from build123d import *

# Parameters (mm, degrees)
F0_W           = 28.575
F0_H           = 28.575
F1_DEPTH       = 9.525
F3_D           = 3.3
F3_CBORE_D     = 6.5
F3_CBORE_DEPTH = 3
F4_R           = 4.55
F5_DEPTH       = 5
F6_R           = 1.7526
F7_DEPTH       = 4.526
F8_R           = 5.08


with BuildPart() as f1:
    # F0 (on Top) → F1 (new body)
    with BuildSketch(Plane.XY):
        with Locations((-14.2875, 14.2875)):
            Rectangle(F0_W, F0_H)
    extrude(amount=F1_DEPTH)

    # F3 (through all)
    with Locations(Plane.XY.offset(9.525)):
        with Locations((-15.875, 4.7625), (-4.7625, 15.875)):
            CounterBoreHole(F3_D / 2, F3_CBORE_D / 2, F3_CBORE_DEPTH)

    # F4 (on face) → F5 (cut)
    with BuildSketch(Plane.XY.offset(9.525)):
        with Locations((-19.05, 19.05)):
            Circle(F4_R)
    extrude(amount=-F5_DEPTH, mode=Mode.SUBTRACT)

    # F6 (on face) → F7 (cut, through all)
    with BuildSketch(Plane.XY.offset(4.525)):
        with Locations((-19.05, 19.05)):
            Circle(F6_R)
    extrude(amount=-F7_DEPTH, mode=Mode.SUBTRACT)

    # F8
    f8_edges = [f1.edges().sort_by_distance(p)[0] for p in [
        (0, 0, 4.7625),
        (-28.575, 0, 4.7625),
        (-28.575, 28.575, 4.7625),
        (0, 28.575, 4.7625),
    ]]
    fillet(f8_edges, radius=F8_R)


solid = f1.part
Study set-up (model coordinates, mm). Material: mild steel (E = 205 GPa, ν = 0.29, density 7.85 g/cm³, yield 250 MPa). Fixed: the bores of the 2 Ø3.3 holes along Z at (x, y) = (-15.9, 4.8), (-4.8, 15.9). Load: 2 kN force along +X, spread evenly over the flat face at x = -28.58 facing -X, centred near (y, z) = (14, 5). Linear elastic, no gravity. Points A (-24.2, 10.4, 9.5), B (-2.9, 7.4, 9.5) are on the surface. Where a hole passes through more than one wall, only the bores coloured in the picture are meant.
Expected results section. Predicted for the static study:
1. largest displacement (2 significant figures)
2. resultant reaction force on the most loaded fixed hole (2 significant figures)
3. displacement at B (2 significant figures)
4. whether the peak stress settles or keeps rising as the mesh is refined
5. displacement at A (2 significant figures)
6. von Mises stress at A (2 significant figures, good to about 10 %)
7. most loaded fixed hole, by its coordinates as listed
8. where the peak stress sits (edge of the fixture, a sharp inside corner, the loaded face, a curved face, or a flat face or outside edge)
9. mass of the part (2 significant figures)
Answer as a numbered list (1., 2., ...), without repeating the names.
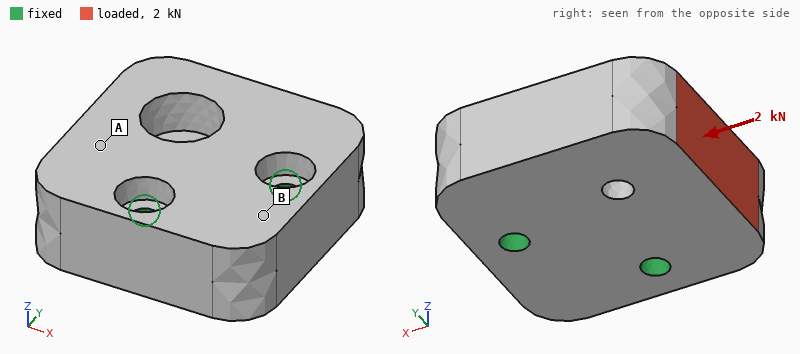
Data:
1. 3.3 µm
2. 1.3 kN
3. 0.51 µm
4. keeps rising
5. 1.7 µm
6. 14 MPa
7. (-4.8, 15.9)
8. edge of the fixture
9. 54 g
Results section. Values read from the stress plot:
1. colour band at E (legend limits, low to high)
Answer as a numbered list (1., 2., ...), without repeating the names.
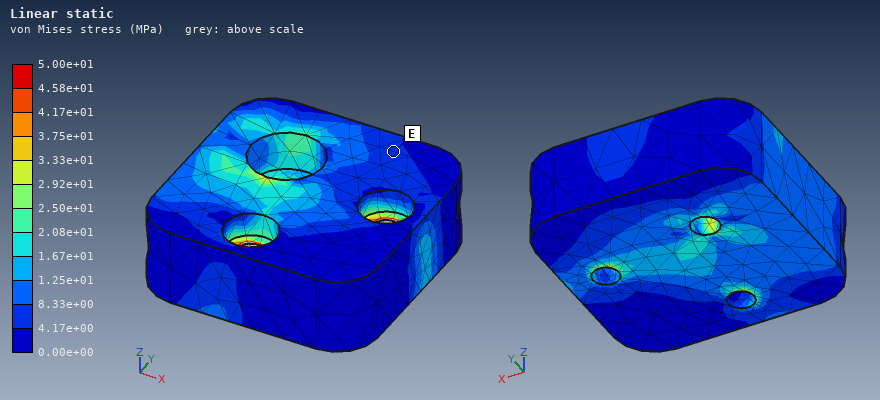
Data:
1. 4.17e+00 to 8.33e+00 MPa
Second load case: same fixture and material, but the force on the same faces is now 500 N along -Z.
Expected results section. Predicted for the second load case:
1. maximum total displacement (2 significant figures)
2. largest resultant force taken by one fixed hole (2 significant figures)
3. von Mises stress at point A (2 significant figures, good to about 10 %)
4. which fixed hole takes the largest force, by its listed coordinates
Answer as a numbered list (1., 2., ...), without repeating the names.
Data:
1. 7.0 µm
2. 490 N
3. 8.5 MPa
4. (-15.9, 4.8)
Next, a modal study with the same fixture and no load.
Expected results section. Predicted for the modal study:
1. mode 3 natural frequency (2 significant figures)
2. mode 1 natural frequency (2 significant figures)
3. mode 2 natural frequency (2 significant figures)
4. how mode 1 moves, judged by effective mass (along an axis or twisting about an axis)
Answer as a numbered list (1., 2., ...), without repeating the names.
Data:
1. 27 kHz
2. 12 kHz
3. 24 kHz
4. along Z
